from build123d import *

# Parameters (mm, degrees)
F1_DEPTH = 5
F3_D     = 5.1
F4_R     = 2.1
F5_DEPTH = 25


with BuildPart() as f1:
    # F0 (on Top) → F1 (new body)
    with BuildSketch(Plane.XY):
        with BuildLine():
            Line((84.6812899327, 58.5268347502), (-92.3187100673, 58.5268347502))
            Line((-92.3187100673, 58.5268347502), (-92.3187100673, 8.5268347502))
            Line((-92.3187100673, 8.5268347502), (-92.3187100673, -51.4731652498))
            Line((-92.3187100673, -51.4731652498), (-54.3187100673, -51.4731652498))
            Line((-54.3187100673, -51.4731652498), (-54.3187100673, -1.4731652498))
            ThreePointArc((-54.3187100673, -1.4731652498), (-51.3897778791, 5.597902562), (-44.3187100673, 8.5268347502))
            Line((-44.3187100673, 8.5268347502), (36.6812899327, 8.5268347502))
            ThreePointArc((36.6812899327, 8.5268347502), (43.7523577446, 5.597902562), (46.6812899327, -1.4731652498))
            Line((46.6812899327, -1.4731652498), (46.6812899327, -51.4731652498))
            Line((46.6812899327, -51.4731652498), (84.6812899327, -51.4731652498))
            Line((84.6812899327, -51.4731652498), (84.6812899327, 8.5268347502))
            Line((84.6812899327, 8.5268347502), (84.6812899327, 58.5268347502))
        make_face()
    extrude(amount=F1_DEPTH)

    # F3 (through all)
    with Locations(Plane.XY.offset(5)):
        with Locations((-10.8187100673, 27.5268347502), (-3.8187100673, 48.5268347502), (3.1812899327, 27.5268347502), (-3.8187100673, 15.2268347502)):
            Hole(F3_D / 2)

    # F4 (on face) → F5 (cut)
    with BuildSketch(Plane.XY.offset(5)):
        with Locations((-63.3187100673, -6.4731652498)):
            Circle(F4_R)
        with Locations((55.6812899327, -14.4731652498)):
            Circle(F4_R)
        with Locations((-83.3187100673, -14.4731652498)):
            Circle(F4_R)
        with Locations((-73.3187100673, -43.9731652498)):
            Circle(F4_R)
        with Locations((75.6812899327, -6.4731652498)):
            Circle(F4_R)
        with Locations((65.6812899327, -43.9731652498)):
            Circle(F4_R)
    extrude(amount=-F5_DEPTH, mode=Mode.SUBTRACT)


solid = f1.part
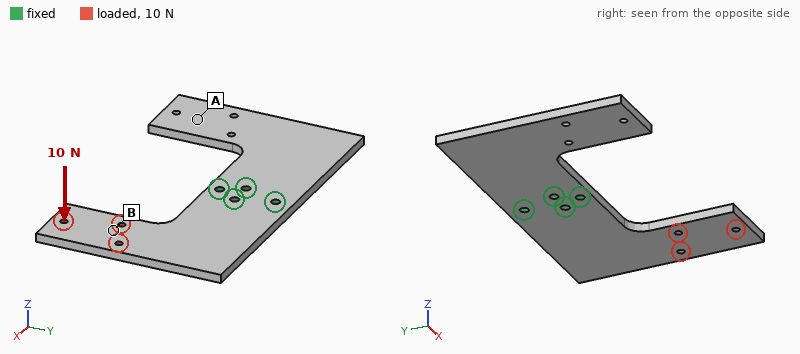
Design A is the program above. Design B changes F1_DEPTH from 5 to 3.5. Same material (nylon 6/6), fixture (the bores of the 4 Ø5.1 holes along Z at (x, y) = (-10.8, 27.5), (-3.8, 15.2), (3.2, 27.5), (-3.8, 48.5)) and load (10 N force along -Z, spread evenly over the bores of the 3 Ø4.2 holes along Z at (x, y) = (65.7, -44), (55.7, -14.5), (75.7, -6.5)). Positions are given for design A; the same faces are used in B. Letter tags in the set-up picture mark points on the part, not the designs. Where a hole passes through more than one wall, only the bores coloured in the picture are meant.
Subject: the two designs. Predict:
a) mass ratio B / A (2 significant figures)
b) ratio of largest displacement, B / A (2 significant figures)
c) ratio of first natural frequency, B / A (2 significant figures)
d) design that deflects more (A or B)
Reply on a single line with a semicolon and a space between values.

0.70; 2.9; 0.71; B
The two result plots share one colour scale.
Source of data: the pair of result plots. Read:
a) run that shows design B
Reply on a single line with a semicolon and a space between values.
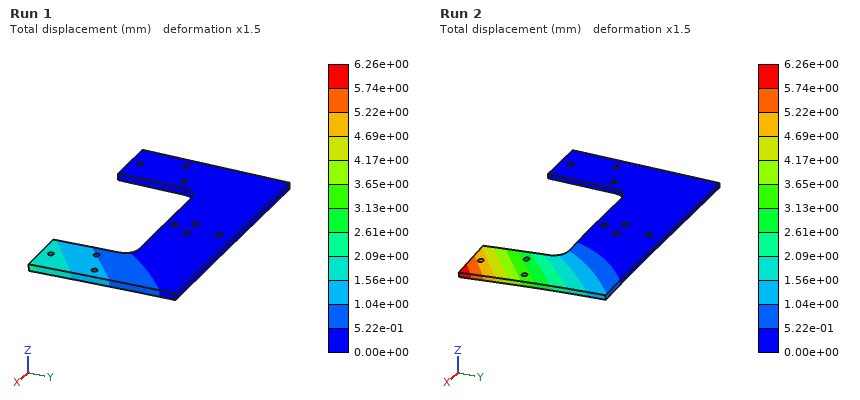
Run 2
